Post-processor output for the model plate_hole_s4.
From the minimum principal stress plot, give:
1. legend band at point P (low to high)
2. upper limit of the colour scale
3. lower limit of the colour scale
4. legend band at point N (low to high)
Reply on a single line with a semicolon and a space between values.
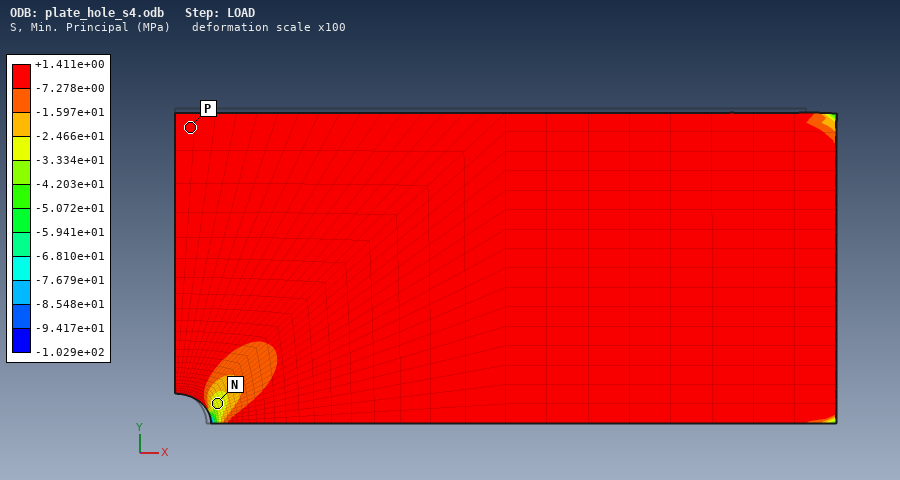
-7.278e+00 to +1.411e+00 MPa; +1.411e+00 MPa; -1.029e+02 MPa; -3.334e+01 to -2.466e+01 MPa
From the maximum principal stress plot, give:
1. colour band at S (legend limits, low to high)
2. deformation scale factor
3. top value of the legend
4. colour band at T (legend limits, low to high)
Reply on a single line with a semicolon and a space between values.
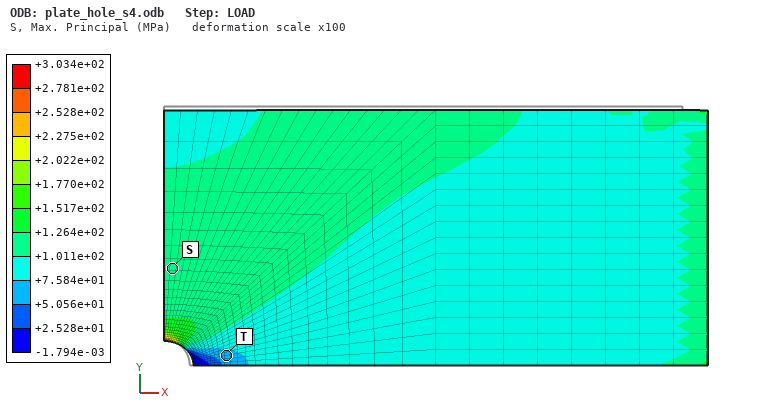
+1.011e+02 to +1.264e+02 MPa; 100; +3.034e+02 MPa; +5.056e+01 to +7.584e+01 MPa
